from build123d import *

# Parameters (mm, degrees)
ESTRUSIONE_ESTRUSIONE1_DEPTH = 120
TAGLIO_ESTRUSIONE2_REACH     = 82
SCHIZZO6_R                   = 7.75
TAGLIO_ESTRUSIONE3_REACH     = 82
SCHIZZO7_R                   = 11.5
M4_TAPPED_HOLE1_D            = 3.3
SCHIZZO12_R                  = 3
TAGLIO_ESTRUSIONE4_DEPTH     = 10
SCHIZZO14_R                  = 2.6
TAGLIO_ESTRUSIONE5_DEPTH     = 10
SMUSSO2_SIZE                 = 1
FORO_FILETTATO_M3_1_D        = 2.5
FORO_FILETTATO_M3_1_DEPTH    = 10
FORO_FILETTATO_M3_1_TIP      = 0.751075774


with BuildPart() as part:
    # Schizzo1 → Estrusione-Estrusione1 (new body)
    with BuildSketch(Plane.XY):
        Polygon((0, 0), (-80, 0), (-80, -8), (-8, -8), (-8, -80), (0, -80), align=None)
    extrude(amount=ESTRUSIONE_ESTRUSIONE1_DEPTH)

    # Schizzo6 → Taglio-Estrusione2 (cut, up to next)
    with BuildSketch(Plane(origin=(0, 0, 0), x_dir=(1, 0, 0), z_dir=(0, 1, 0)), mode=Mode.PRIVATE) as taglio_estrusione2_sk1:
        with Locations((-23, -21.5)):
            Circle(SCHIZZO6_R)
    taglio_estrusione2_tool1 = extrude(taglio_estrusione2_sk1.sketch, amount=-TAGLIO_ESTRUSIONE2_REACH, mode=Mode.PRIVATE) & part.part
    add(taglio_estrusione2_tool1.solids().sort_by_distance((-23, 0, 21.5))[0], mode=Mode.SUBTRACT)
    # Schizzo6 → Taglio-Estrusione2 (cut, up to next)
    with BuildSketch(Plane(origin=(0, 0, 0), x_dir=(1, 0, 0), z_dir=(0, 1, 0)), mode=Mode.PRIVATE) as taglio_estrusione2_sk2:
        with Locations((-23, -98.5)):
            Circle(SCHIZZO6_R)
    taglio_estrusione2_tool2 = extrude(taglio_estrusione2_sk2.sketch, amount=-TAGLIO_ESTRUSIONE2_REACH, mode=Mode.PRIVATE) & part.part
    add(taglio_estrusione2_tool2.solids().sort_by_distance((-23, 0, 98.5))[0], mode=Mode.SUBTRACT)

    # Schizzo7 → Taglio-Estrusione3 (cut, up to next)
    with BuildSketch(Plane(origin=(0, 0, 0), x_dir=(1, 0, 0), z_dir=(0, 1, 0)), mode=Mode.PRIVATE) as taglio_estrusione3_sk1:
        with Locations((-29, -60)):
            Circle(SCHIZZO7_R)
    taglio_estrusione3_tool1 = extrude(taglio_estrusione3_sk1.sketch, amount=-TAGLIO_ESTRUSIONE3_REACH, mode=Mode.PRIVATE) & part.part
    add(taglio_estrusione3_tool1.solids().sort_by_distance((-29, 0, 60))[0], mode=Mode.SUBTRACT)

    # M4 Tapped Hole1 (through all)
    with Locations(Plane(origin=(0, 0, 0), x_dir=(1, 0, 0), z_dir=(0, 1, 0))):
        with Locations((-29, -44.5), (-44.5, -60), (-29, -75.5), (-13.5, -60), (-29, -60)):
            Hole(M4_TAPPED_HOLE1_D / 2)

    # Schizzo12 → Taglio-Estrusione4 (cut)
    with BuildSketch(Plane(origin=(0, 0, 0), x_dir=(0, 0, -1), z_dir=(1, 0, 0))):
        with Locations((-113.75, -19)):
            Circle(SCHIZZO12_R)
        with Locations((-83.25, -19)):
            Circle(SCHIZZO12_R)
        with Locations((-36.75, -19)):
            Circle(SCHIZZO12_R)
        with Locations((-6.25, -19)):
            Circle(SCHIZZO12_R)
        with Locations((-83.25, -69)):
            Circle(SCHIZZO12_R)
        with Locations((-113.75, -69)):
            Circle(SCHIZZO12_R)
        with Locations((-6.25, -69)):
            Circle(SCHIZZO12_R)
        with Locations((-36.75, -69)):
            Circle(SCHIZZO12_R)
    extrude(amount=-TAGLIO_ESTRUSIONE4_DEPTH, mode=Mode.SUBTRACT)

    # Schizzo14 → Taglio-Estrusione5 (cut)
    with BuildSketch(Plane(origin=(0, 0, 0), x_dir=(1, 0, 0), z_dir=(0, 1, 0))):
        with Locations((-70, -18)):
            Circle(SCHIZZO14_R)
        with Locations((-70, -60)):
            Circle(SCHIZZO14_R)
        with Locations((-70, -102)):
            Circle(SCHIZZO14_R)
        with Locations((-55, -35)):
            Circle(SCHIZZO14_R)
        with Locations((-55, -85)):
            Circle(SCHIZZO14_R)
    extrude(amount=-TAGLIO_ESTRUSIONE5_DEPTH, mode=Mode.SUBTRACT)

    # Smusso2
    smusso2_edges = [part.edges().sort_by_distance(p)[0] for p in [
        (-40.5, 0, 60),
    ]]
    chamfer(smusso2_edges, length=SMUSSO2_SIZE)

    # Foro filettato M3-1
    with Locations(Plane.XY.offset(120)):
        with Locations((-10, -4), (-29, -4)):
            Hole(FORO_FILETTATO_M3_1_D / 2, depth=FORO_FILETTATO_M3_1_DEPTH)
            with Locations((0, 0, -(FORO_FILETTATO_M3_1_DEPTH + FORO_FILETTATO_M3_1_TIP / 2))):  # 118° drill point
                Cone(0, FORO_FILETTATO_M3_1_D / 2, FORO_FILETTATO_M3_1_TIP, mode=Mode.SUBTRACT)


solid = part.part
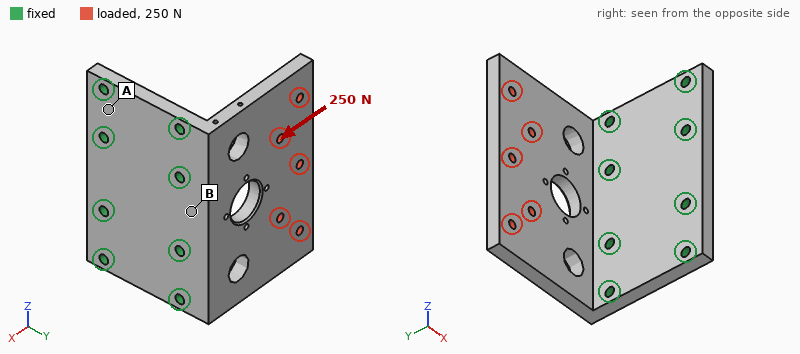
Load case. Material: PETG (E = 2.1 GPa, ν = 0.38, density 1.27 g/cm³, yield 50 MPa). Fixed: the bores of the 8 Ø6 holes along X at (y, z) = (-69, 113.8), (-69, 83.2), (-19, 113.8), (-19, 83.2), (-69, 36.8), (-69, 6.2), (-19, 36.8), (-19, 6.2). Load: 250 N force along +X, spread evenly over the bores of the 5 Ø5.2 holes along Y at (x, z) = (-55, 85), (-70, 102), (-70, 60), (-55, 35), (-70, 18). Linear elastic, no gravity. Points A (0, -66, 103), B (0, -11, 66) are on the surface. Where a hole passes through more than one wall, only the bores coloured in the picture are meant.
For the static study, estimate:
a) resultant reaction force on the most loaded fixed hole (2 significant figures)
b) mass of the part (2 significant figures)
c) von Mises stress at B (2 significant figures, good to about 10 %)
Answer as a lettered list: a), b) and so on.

a) 79 N
b) 170 g
c) 0.72 MPa
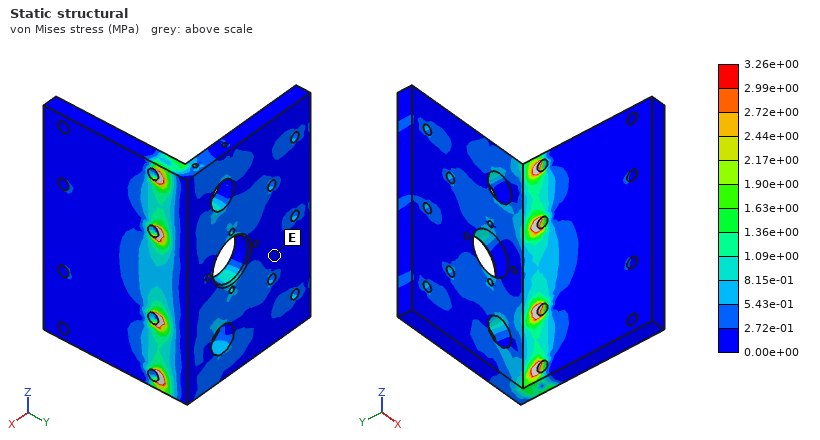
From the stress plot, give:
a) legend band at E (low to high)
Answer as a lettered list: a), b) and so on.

a) 0.00e+00 to 2.72e-01 MPa
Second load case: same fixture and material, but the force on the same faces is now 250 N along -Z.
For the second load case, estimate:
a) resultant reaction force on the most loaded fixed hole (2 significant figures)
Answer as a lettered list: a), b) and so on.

a) 130 N
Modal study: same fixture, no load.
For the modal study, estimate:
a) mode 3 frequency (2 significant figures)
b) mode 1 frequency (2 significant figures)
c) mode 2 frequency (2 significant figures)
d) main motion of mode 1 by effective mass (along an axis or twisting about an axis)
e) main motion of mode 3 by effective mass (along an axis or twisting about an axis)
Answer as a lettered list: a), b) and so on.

a) 1000 Hz
b) 210 Hz
c) 410 Hz
d) along Y
e) along Z
